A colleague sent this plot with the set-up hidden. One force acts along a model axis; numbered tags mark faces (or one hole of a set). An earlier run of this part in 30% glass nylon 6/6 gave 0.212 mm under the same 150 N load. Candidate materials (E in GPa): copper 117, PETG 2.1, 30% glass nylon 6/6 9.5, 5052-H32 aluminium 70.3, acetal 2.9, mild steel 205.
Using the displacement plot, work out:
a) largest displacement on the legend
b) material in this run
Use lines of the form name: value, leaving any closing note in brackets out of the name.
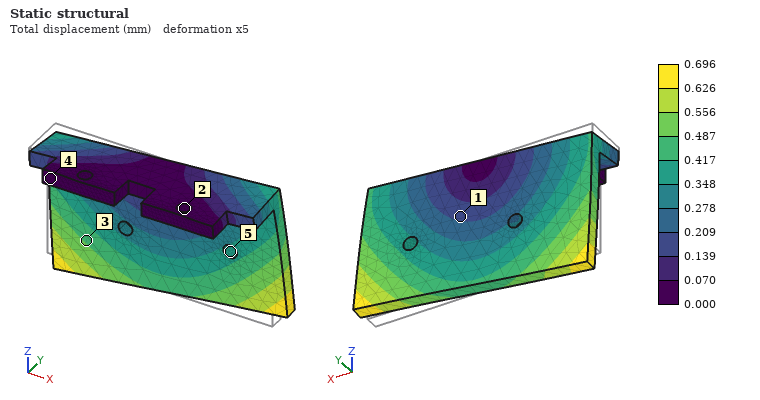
largest displacement on the legend: 0.696 mm
material in this run: acetal
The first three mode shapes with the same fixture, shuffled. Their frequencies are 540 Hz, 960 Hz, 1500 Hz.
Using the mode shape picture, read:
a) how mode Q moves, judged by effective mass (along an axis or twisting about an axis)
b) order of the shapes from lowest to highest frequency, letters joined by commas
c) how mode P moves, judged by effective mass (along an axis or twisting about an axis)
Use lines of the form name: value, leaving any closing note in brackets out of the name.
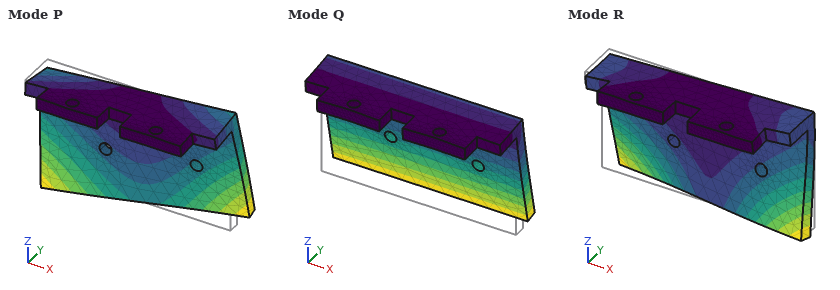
how mode Q moves, judged by effective mass: along Y
order of the shapes from lowest to highest frequency, letters joined by commas: Q, P, R
how mode P moves, judged by effective mass: along X
